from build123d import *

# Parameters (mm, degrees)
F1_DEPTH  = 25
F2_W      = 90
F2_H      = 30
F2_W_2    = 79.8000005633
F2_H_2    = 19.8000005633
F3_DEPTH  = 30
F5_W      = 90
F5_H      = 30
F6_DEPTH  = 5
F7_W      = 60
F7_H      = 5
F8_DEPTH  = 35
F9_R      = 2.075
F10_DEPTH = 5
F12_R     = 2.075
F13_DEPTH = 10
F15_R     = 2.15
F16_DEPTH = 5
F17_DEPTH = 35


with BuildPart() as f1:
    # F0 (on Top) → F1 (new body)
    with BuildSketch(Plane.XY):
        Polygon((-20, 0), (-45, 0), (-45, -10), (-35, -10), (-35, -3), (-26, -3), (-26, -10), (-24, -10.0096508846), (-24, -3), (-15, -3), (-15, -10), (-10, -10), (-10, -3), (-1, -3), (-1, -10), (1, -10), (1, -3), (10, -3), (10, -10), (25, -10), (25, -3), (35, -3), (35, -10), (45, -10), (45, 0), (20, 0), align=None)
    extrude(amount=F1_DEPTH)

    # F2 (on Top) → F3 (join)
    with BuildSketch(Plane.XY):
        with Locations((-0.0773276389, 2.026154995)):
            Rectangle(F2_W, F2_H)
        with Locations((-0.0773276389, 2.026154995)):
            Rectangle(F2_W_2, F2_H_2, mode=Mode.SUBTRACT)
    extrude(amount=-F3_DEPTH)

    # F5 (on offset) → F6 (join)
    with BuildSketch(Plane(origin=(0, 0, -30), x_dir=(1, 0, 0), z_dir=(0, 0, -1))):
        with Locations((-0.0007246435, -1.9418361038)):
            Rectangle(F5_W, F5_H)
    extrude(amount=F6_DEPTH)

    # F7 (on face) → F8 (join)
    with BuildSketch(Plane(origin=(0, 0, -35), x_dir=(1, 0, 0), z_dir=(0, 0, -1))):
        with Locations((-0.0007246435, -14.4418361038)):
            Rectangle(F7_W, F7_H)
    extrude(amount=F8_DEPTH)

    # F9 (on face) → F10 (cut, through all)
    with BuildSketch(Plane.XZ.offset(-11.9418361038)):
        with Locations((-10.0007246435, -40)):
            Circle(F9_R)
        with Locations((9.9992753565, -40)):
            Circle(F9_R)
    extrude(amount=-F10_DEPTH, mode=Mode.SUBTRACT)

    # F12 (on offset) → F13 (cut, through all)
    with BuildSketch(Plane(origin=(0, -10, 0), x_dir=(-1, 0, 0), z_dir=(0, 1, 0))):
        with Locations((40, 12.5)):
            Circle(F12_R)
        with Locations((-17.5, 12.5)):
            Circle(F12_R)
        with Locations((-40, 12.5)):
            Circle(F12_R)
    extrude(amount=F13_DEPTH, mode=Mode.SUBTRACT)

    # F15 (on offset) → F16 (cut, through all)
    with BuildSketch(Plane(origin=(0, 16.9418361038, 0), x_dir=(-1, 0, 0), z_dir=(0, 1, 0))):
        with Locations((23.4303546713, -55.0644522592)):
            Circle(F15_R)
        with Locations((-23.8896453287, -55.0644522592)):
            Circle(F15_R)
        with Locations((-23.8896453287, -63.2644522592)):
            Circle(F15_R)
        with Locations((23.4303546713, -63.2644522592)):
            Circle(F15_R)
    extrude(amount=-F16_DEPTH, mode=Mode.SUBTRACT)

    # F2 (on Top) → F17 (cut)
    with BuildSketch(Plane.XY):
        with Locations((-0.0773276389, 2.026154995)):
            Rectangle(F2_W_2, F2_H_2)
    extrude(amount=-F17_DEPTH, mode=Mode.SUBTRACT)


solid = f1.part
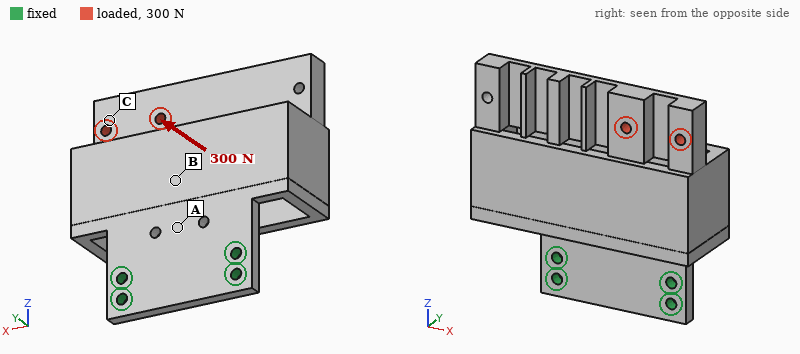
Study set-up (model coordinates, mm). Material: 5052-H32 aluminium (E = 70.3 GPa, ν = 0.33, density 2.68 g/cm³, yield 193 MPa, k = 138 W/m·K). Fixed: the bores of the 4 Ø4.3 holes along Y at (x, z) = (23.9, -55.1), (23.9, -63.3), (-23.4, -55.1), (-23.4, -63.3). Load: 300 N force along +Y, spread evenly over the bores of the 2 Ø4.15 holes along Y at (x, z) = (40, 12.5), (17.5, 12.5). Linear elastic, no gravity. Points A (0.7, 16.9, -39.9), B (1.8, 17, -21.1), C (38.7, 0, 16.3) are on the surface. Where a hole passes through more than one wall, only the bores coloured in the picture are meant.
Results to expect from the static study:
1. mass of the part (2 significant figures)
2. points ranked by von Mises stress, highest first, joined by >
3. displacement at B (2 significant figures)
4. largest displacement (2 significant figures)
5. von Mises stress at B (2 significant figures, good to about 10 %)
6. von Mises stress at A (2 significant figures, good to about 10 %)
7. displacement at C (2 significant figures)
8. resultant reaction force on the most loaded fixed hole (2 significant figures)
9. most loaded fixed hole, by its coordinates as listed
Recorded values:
170 g
A > B > C
0.25 mm
1.1 mm
25 MPa
57 MPa
0.92 mm
760 N
(23.9, -55.1)
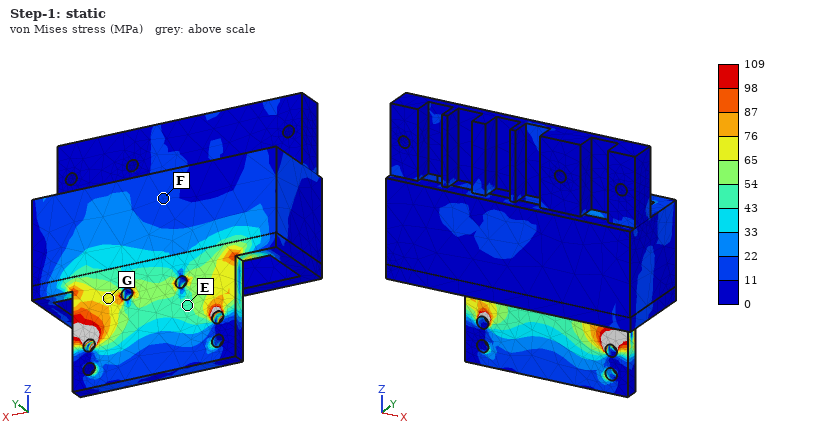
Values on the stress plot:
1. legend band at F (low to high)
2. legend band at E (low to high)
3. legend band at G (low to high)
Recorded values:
11 to 22 MPa
43 to 54 MPa
65 to 76 MPa
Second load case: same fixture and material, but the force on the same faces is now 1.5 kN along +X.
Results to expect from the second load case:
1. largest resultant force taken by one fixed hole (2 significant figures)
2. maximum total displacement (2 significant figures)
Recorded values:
2.0 kN
0.42 mm
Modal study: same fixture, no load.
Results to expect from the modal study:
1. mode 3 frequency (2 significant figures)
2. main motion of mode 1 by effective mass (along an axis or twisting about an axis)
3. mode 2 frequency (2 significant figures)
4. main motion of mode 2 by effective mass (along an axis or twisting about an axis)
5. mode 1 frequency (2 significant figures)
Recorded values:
1700 Hz
along Y
790 Hz
along X
370 Hz
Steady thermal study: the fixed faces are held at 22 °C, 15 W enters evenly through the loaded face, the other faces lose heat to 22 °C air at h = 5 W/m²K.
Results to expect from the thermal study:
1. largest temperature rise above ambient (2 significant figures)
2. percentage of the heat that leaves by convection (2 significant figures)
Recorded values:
35 K
17 %
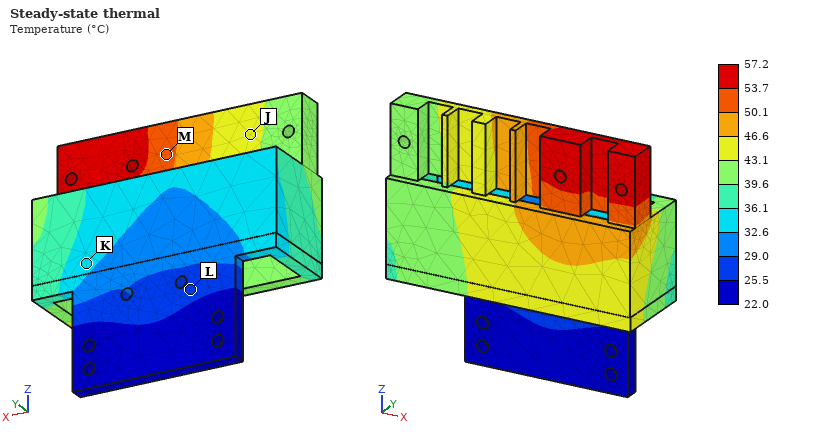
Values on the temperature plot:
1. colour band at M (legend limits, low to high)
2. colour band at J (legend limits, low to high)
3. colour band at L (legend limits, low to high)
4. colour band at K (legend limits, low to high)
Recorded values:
50.1 to 53.7 °C
43.1 to 46.6 °C
25.5 to 29.0 °C
32.6 to 36.1 °C
